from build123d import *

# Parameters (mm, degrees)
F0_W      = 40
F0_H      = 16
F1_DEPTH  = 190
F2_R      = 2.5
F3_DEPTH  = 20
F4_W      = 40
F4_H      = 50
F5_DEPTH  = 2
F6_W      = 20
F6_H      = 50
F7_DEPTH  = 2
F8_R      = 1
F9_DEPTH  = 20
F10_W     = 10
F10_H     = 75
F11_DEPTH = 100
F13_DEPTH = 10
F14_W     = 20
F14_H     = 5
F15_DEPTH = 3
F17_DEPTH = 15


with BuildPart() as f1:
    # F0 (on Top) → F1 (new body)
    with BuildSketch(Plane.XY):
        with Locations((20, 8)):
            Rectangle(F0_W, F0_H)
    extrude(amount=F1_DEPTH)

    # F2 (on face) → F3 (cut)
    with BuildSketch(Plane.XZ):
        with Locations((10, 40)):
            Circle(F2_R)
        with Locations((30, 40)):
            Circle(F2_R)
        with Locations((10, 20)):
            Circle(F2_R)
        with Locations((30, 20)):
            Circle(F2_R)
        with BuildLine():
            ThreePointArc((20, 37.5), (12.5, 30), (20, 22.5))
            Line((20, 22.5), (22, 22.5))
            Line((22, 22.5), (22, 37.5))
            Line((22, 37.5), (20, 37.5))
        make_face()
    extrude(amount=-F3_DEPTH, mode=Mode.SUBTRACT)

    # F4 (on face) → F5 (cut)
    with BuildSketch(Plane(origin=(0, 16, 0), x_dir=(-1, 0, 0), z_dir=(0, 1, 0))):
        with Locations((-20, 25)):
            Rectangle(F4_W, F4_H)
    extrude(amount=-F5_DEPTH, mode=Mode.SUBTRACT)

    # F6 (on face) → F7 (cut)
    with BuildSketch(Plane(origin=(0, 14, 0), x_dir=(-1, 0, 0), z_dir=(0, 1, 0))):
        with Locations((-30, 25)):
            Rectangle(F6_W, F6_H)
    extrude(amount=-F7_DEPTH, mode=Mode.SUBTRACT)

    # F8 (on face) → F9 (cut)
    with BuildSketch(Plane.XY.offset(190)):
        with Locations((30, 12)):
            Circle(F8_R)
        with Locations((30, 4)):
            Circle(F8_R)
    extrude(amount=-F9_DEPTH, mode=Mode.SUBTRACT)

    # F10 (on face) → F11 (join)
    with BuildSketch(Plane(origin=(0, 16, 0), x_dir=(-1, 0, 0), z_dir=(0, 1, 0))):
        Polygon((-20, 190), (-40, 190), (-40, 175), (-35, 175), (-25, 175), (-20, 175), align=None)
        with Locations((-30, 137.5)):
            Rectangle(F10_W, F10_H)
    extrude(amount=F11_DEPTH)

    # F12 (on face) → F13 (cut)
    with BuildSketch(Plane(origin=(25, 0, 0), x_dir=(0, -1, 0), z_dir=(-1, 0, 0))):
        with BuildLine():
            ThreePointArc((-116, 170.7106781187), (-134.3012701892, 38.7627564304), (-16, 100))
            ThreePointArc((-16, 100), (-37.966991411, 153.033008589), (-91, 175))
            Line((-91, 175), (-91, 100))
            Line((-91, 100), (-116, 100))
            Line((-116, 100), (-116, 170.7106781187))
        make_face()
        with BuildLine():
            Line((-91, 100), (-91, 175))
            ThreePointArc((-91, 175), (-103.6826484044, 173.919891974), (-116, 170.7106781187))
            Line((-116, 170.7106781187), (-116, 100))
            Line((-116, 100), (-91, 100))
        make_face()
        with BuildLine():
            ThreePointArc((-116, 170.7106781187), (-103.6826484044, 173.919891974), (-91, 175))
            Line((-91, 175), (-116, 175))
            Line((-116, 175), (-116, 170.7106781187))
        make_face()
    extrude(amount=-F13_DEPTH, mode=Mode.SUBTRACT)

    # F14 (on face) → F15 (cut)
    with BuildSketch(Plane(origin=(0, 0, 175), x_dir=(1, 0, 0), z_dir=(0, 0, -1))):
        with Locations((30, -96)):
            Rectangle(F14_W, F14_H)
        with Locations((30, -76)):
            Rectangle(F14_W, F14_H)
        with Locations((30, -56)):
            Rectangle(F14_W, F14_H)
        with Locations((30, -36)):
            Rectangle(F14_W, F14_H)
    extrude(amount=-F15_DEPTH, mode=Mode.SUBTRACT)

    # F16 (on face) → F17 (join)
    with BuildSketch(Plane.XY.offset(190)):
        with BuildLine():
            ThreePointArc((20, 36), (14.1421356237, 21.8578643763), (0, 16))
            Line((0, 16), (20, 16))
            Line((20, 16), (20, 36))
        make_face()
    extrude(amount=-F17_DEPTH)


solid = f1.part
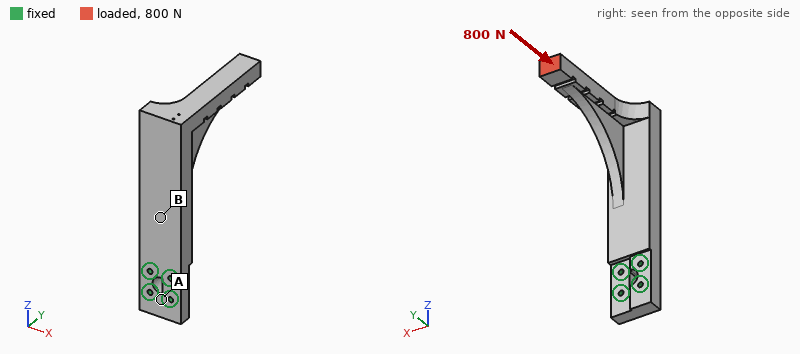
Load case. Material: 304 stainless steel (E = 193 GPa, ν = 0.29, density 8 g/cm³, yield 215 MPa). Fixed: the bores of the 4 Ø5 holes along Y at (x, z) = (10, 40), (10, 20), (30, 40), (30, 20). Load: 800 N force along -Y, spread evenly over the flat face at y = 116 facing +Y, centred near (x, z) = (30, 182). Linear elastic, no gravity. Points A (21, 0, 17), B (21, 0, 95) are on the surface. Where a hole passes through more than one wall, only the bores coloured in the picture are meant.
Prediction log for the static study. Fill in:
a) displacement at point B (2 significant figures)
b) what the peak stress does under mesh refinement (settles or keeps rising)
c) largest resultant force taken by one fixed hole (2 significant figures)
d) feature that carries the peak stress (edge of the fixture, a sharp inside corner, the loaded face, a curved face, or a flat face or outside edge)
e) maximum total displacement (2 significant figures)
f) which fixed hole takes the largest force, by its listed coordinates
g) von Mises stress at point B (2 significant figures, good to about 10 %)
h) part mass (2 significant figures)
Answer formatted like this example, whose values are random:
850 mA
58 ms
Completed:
0.086 mm
keeps rising
1.0 kN
edge of the fixture
0.53 mm
(30, 40)
41 MPa
1.2 kg
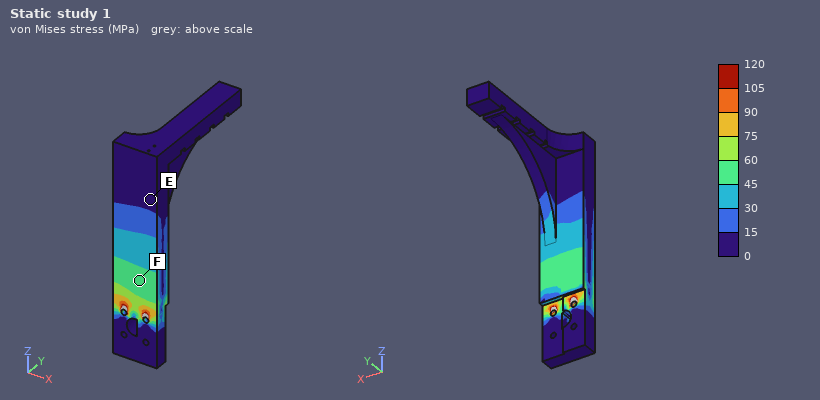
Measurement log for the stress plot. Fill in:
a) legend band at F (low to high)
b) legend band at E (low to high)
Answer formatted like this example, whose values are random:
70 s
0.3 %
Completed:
45 to 60 MPa
0 to 15 MPa
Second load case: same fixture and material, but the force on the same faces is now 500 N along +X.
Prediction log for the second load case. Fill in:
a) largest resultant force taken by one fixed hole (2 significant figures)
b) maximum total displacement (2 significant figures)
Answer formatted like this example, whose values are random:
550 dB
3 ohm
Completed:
3.0 kN
0.35 mm
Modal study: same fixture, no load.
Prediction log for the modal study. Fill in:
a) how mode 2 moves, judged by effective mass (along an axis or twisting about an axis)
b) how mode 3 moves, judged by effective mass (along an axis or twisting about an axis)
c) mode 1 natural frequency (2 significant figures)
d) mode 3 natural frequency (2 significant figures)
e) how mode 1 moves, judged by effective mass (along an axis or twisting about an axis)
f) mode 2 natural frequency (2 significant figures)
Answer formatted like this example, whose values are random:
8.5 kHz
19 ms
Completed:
along X
along X
300 Hz
1200 Hz
along Y
600 Hz
